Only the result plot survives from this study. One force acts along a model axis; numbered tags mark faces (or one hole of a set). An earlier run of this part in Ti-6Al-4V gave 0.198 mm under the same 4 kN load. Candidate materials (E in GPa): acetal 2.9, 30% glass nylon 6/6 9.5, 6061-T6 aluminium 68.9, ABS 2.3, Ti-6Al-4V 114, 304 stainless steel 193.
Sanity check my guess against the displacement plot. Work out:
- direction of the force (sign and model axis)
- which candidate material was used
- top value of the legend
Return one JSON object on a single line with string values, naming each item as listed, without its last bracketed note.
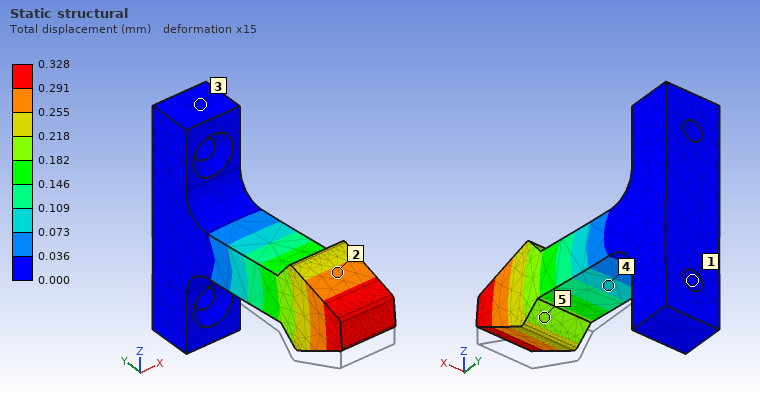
{"direction of the force": "+Z", "which candidate material was used": "6061-T6 aluminium", "top value of the legend": "0.328 mm"}
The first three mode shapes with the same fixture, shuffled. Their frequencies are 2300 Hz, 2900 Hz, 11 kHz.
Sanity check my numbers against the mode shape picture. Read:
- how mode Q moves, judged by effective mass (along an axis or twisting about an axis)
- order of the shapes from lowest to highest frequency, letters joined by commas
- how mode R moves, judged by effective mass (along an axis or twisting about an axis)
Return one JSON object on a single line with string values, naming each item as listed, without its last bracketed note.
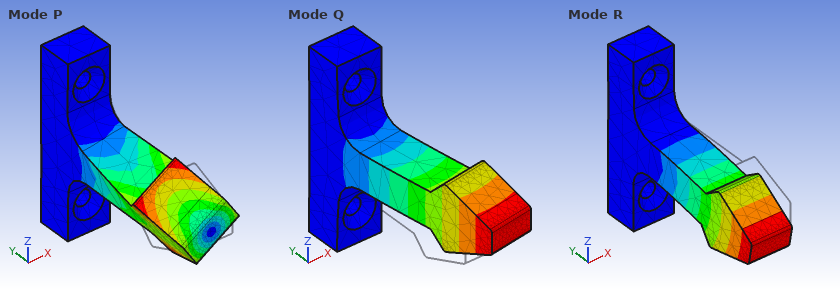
{"how mode Q moves, judged by effective mass": "along X", "order of the shapes from lowest to highest frequency, letters joined by commas": "Q, R, P", "how mode R moves, judged by effective mass": "along Z"}
